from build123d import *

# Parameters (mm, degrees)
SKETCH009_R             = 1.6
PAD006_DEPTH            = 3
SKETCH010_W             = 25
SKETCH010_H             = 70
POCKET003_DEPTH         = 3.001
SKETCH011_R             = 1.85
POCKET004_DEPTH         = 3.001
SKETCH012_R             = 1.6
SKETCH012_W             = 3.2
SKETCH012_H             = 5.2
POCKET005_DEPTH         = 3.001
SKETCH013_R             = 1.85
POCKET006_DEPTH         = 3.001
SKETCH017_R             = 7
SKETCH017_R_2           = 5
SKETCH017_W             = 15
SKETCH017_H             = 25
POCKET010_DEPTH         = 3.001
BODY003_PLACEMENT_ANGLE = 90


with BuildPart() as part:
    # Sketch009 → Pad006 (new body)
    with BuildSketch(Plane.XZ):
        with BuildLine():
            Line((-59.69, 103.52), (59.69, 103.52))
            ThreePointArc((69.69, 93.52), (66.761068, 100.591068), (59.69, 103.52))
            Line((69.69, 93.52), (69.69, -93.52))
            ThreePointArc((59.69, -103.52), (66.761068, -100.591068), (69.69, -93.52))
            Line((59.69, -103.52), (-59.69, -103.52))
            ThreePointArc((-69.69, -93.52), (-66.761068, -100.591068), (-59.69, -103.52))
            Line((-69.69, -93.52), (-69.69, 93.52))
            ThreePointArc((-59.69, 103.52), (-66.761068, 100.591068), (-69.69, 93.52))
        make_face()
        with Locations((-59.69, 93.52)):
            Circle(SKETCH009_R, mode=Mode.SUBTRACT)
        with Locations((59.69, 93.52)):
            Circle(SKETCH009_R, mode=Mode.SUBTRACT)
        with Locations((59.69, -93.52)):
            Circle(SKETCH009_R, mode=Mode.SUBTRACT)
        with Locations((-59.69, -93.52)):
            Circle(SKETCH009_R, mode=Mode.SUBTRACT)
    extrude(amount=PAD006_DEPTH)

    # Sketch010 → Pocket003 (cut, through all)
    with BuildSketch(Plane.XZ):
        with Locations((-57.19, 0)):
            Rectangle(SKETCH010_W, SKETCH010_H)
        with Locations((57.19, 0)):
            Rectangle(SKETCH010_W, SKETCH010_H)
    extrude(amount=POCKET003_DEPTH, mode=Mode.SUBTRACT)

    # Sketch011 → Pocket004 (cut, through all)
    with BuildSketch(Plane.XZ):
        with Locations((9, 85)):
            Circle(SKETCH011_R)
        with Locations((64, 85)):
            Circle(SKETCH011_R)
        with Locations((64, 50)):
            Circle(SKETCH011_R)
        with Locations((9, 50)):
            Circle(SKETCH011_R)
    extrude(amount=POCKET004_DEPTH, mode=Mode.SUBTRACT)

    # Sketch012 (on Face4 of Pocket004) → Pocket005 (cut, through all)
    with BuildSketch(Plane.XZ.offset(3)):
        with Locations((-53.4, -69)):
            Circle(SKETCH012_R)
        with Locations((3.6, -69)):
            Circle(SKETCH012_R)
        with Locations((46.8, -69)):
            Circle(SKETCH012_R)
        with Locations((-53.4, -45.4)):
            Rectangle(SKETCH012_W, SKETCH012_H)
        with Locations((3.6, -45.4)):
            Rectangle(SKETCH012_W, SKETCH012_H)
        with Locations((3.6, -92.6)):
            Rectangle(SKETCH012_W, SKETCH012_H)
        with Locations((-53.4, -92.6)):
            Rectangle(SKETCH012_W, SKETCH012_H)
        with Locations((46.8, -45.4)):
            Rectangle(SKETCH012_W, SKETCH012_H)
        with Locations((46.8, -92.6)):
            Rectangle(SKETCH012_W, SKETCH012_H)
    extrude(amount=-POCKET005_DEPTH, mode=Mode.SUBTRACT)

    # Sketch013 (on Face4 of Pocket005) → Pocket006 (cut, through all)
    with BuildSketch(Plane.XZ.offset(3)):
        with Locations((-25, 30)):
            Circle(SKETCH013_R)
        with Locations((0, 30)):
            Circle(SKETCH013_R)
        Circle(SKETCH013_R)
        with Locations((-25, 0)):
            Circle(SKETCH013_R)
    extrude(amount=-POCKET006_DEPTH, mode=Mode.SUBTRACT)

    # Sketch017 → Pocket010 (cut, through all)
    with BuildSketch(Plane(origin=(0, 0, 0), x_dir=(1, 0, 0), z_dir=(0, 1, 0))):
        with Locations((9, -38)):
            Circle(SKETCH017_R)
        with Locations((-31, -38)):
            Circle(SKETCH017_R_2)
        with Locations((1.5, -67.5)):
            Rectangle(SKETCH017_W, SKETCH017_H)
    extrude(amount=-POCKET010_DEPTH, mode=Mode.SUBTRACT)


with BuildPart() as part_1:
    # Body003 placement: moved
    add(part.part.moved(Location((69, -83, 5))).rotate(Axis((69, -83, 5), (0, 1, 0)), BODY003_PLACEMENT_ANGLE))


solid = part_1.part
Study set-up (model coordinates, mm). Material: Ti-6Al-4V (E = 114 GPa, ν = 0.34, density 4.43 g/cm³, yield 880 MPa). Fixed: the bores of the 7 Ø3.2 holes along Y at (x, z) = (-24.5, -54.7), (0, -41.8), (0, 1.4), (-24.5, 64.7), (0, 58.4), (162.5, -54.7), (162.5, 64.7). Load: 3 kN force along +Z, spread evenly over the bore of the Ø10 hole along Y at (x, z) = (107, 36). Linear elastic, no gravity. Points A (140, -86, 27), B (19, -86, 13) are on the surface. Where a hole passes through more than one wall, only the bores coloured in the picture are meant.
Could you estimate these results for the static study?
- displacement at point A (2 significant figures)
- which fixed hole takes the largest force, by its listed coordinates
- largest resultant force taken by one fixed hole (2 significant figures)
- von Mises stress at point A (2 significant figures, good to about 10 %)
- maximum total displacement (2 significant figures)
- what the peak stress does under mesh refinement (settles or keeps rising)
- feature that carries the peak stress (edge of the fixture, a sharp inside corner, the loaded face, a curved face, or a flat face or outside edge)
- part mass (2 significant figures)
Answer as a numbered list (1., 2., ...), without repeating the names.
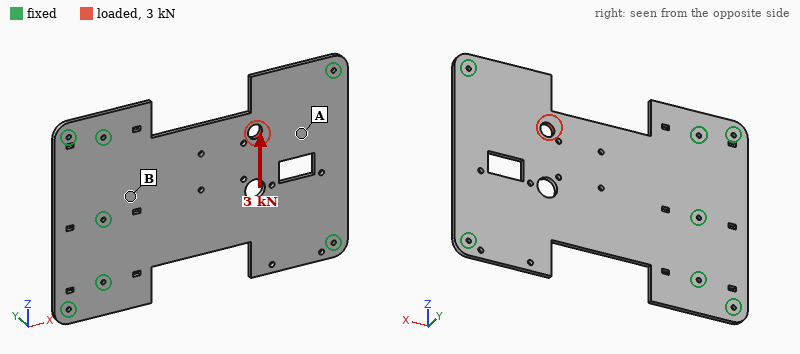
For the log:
1. 10 µm
2. (162.5, 64.7)
3. 1.3 kN
4. 18 MPa
5. 23 µm
6. keeps rising
7. edge of the fixture
8. 320 g
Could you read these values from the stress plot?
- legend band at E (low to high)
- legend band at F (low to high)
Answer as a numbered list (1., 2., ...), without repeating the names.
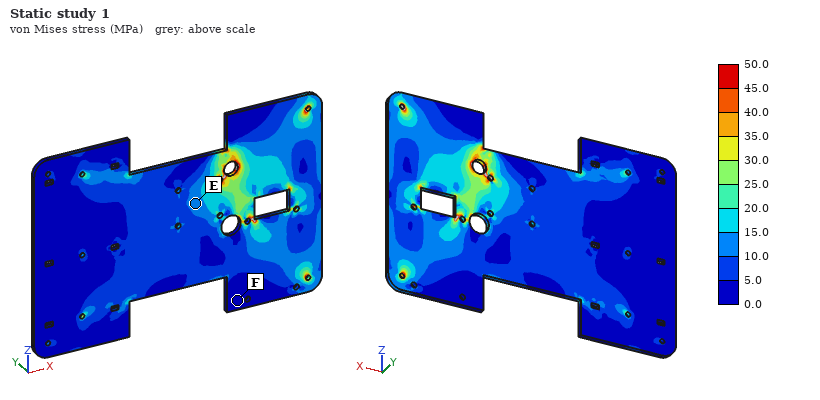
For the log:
1. 10.0 to 15.0 MPa
2. 0.0 to 5.0 MPa
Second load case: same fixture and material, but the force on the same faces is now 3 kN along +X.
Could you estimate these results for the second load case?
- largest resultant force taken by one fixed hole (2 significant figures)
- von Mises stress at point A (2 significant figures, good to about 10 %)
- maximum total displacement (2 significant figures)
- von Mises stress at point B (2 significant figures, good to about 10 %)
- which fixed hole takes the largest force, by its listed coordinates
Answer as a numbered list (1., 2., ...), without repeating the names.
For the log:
1. 1.1 kN
2. 7.9 MPa
3. 13 µm
4. 6.6 MPa
5. (162.5, 64.7)
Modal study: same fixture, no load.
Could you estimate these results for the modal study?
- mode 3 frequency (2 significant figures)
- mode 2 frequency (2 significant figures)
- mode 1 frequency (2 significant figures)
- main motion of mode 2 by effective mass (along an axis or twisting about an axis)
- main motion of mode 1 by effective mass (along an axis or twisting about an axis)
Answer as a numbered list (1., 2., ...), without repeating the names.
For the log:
1. 1100 Hz
2. 880 Hz
3. 500 Hz
4. twisting about X
5. along Y
